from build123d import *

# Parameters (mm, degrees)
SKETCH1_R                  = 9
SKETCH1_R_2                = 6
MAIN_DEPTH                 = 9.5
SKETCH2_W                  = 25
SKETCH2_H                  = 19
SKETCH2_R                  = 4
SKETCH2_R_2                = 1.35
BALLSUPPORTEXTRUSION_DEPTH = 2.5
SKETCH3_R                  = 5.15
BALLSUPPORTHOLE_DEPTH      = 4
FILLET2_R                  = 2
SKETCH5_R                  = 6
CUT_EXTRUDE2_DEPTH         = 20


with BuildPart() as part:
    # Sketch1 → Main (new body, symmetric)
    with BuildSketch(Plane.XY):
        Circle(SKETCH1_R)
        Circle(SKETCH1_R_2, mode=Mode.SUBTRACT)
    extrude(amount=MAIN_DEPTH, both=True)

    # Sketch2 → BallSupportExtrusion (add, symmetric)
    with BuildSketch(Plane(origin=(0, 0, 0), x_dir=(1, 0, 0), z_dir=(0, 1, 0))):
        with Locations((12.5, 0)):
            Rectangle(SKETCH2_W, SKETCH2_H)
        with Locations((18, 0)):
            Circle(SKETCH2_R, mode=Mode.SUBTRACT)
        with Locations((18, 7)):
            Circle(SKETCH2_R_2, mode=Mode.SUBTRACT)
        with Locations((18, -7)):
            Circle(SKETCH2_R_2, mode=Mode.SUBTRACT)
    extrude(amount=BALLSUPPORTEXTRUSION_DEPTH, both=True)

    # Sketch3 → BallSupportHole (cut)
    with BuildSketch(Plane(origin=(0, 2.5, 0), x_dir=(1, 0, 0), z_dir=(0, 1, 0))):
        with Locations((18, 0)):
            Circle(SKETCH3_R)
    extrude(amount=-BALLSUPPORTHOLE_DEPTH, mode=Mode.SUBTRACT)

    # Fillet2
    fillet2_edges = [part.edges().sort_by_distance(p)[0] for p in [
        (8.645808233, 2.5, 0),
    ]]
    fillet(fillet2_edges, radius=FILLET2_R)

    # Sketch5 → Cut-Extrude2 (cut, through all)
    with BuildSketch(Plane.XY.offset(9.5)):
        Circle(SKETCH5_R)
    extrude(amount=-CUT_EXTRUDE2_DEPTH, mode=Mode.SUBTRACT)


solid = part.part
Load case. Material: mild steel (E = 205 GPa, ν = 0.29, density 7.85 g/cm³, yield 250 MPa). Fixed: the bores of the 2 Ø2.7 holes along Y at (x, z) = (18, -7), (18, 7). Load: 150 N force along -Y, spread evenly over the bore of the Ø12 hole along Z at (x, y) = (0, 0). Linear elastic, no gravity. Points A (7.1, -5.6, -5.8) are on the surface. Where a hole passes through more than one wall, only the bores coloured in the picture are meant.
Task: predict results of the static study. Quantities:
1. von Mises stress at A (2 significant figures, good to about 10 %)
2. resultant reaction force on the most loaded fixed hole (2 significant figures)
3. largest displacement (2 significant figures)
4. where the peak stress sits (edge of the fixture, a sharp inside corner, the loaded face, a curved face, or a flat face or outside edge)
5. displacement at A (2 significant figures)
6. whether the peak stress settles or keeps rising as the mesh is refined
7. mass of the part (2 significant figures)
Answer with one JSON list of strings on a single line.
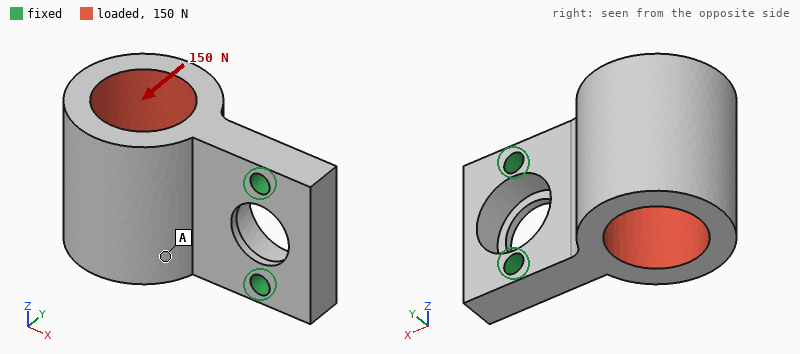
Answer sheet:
["7.9 MPa", "75 N", "18 µm", "edge of the fixture", "6.3 µm", "keeps rising", "30 g"]
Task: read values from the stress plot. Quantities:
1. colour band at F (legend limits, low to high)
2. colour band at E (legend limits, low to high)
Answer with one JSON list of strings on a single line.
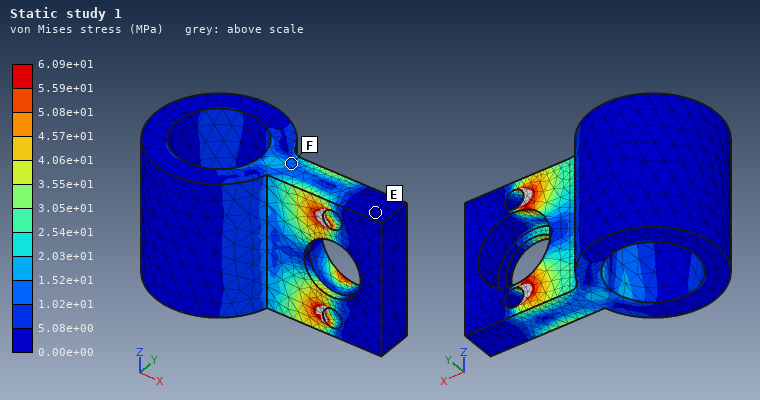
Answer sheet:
["1.02e+01 to 1.52e+01 MPa", "0.00e+00 to 5.08e+00 MPa"]
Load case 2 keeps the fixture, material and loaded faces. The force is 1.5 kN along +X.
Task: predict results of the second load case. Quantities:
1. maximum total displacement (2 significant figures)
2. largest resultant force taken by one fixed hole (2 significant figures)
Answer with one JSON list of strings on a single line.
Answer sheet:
["5.8 µm", "770 N"]
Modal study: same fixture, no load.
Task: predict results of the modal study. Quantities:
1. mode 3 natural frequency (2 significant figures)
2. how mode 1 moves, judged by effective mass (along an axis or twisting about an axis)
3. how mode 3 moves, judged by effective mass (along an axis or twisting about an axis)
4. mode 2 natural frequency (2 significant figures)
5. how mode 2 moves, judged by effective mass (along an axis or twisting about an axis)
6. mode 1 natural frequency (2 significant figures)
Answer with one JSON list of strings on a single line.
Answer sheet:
["14 kHz", "along Y", "twisting about X", "11 kHz", "along Z", "3500 Hz"]
